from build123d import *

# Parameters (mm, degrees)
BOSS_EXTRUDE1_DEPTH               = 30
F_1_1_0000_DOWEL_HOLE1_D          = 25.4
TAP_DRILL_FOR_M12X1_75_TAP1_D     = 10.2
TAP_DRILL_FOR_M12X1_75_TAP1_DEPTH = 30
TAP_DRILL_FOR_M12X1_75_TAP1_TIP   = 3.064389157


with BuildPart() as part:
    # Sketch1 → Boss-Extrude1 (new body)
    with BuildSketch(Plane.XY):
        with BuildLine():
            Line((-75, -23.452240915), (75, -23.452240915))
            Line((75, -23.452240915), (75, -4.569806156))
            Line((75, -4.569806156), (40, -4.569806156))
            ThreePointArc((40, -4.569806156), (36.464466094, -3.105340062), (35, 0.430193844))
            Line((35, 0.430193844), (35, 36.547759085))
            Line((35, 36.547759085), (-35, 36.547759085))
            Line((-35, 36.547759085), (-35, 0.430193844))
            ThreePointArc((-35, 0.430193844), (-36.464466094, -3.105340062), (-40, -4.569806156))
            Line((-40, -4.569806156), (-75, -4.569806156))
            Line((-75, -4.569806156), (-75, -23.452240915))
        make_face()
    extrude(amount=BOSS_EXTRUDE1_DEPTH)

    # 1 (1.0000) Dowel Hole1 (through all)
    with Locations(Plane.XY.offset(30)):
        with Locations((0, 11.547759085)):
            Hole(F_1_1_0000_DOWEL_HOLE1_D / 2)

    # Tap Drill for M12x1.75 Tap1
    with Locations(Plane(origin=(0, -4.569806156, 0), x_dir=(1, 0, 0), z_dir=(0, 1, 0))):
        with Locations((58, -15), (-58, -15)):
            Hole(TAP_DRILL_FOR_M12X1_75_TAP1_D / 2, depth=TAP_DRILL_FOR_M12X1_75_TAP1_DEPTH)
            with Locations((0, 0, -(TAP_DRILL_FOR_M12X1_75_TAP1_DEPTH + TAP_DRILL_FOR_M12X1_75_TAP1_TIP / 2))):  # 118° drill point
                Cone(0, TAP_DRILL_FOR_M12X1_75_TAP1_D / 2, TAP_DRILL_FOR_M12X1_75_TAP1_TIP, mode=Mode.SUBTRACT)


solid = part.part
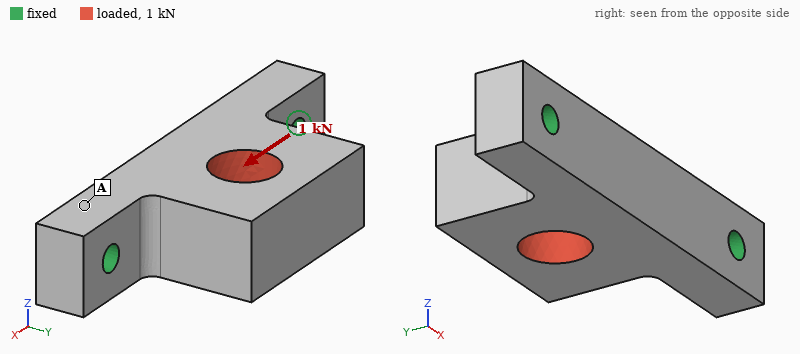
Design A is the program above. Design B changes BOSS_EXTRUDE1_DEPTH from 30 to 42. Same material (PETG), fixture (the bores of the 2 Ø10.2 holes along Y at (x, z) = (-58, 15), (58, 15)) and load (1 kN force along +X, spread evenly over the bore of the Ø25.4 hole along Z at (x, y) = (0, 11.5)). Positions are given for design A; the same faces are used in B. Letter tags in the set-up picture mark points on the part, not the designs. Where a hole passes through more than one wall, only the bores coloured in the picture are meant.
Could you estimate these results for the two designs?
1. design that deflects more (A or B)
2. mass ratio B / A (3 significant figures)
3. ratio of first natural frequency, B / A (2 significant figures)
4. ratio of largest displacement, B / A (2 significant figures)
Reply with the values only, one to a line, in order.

A
1.41
1.0
0.81
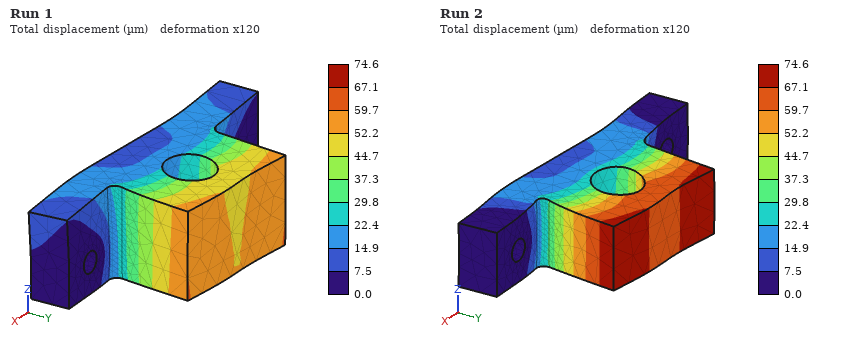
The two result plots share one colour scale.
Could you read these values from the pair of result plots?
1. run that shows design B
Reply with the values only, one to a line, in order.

Run 1
